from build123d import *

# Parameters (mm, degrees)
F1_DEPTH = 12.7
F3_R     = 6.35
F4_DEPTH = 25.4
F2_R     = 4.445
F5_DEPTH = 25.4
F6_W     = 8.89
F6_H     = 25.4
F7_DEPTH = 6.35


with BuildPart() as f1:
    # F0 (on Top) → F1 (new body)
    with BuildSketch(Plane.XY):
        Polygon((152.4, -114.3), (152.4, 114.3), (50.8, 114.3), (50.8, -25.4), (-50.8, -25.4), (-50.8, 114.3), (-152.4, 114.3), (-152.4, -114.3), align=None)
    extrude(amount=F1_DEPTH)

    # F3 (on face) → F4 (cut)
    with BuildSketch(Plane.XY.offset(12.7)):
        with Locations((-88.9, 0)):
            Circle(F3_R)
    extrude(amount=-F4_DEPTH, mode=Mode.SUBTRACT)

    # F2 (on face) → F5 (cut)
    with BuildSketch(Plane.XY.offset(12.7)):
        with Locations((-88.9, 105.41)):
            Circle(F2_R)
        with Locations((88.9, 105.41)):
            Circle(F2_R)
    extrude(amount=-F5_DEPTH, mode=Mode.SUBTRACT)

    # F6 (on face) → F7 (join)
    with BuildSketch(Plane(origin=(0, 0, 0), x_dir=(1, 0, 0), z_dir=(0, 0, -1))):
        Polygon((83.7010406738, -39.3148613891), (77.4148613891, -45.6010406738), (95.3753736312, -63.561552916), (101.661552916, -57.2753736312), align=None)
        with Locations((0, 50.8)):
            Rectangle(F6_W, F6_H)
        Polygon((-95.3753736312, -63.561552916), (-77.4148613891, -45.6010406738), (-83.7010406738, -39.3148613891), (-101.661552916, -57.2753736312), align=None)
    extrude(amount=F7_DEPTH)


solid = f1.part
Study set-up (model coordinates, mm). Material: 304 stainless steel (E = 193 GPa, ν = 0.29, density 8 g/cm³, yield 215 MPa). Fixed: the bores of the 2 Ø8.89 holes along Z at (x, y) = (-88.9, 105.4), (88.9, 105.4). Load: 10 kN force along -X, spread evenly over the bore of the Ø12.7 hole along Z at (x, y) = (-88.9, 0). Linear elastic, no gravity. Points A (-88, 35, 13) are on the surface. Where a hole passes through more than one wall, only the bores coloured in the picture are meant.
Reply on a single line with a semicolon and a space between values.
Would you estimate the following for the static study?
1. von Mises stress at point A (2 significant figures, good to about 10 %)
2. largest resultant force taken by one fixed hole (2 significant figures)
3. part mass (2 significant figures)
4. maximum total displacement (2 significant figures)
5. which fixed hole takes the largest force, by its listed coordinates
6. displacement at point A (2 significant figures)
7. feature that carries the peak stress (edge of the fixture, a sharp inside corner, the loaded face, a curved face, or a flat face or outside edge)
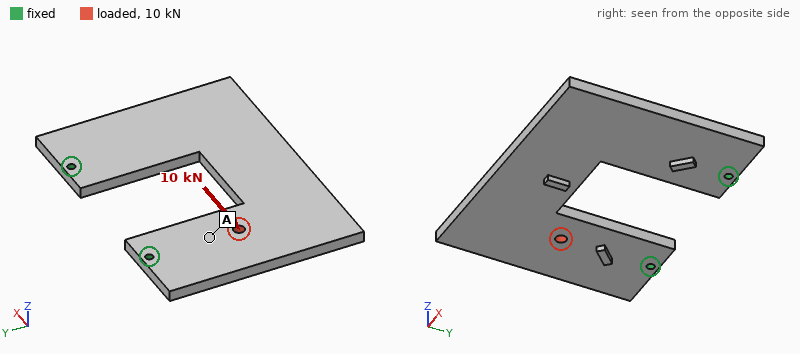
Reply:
15 MPa; 8.2 kN; 5.6 kg; 73 µm; (-88.9, 105.4); 37 µm; edge of the fixture
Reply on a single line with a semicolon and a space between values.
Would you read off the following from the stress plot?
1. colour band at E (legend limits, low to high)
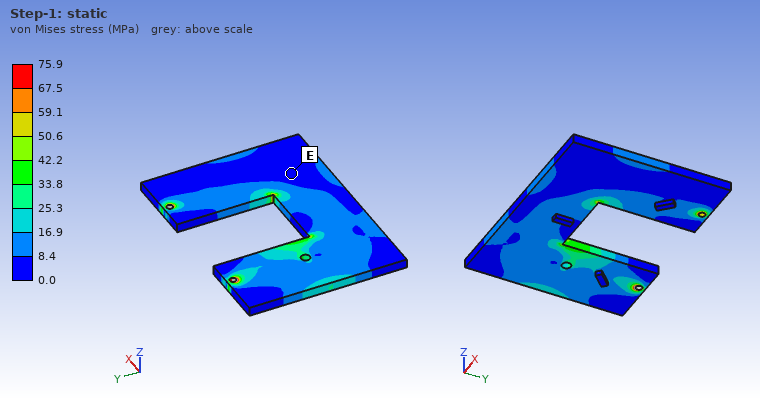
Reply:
0.0 to 8.4 MPa
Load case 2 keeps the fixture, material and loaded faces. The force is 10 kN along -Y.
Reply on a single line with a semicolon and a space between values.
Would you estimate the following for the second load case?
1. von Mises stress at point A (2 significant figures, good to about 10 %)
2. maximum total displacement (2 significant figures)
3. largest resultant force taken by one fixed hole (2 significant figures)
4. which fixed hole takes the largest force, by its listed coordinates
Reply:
13 MPa; 13 µm; 9.9 kN; (-88.9, 105.4)
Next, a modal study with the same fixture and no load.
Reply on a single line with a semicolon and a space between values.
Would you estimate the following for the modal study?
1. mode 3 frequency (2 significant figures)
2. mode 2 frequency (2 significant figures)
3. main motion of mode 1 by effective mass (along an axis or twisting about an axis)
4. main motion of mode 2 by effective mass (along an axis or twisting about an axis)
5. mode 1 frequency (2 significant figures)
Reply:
780 Hz; 310 Hz; along Z; twisting about Y; 150 Hz
